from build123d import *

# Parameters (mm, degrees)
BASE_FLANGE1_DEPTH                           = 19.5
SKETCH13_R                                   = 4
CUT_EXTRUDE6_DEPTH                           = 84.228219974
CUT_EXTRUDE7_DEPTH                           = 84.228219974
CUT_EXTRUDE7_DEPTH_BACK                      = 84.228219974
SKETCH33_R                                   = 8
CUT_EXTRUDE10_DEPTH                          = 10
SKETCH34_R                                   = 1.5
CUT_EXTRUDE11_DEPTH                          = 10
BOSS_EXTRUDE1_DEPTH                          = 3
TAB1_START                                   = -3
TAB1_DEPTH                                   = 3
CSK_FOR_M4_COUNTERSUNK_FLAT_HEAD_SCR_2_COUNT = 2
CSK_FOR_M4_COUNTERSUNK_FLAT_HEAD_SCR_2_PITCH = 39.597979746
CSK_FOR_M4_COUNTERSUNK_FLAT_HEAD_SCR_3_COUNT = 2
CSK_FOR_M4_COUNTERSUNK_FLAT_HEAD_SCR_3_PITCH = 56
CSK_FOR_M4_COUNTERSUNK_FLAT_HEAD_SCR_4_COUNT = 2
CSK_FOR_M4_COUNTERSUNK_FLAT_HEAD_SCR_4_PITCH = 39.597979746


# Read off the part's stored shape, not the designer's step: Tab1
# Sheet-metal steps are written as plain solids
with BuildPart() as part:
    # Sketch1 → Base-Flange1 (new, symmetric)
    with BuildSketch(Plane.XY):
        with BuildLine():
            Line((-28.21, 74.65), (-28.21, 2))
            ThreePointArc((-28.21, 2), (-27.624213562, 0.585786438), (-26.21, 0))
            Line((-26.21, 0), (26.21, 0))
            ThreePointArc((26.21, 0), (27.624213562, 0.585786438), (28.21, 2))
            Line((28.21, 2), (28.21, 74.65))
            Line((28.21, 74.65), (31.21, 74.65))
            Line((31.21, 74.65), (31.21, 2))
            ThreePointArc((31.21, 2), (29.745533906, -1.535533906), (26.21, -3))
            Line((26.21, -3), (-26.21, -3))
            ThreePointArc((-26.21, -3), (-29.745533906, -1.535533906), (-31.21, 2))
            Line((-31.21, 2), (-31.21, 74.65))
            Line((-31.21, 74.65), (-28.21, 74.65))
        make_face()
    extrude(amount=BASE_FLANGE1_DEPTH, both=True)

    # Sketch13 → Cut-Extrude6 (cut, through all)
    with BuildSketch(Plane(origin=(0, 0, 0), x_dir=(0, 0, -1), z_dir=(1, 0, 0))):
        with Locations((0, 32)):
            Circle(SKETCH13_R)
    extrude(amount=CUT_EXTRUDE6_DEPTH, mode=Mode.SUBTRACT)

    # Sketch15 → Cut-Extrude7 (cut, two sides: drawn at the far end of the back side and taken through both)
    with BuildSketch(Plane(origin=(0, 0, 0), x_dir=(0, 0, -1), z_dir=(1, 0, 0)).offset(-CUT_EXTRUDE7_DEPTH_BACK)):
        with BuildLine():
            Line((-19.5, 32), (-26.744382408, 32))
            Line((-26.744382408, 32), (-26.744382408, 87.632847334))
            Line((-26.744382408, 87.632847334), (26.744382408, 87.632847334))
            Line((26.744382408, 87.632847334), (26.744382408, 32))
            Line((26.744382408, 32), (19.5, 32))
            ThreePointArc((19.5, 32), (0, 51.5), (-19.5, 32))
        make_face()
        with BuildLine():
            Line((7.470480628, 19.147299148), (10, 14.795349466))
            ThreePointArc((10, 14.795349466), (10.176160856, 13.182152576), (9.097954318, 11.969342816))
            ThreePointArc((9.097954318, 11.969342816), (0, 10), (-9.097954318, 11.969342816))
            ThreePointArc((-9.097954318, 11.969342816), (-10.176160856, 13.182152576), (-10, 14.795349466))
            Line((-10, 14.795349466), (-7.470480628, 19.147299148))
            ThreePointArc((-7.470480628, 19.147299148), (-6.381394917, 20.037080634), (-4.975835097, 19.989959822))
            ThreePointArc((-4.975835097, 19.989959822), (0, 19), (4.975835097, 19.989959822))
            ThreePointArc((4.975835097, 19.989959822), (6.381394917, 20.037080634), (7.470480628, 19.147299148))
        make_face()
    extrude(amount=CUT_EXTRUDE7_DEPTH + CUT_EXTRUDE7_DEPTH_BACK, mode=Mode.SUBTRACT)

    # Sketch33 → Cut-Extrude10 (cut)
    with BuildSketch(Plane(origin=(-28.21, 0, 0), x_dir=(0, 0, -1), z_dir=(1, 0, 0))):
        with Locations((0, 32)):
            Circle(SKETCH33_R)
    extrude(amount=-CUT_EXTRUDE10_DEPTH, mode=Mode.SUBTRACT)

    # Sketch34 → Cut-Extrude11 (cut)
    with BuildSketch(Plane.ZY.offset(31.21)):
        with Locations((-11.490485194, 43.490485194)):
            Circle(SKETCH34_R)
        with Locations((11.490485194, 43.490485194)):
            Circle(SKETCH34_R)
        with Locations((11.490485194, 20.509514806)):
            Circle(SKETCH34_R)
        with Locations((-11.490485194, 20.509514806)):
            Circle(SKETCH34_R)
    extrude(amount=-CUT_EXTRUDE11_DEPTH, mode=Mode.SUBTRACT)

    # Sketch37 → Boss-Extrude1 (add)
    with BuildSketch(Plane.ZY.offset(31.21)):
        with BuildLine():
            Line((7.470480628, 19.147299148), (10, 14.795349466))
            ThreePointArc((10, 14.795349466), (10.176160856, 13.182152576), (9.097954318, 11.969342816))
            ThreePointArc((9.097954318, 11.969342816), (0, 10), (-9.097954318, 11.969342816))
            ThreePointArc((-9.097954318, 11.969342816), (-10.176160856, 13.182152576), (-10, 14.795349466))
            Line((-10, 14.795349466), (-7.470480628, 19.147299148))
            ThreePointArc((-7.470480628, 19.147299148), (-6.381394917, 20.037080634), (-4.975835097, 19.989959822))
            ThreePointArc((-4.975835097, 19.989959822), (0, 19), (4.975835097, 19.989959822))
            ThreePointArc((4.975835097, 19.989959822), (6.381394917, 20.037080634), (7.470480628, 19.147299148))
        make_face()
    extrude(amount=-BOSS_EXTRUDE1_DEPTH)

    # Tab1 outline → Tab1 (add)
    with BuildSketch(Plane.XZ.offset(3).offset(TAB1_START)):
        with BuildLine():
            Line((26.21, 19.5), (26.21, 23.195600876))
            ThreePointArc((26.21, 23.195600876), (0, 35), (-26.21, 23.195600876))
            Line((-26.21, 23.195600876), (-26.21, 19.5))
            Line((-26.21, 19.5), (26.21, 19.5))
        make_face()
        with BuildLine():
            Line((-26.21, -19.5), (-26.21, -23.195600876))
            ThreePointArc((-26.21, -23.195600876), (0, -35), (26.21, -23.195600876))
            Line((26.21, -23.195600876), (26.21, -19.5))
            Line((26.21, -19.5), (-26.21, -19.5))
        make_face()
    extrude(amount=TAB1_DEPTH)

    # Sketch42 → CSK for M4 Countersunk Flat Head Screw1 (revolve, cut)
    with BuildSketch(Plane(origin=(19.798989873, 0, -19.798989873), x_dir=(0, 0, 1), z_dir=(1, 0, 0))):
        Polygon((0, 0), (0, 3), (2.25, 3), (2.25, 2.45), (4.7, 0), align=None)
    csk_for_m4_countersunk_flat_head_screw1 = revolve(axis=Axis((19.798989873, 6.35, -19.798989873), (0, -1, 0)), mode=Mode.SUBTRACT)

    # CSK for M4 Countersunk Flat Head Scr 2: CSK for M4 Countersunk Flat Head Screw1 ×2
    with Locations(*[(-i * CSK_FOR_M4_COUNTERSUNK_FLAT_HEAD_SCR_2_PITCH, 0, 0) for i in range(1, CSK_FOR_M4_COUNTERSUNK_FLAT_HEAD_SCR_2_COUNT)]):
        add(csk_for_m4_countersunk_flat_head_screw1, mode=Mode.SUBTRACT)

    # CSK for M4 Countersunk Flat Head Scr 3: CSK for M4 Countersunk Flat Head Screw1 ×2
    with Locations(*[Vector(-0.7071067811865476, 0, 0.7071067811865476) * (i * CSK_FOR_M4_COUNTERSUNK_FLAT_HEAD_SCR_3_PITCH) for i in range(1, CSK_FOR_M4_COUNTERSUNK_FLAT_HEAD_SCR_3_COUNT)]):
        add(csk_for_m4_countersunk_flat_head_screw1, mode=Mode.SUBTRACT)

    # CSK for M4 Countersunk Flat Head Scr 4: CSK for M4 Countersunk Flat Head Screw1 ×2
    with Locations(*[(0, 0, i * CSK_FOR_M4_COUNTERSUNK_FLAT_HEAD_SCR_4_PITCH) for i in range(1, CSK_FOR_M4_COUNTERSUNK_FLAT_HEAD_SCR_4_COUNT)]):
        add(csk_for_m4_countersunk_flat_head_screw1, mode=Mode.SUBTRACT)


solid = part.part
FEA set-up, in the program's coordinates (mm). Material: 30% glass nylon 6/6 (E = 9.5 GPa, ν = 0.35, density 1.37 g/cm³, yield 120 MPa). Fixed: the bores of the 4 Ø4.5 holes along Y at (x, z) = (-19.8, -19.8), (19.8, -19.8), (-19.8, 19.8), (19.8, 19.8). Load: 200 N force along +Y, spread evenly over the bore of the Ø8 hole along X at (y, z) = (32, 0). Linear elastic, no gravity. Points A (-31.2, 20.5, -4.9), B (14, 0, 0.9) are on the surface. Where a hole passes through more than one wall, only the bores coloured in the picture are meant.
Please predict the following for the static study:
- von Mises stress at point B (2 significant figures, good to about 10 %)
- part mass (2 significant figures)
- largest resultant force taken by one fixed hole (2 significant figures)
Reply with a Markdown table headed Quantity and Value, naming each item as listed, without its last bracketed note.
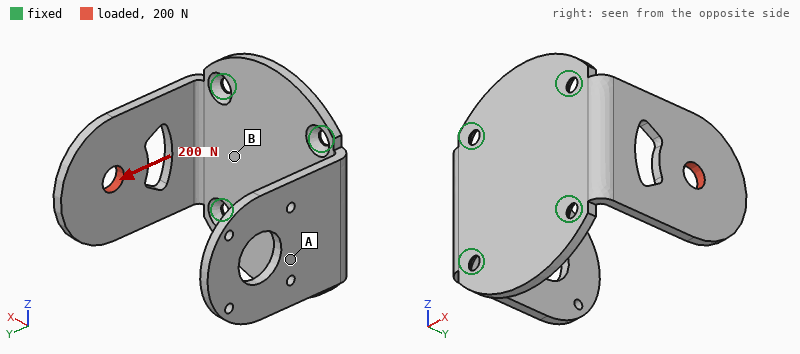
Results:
| Quantity | Value |
|---|---|
| von Mises stress at point B | 11 MPa |
| part mass | 27 g |
| largest resultant force taken by one fixed hole | 200 N |
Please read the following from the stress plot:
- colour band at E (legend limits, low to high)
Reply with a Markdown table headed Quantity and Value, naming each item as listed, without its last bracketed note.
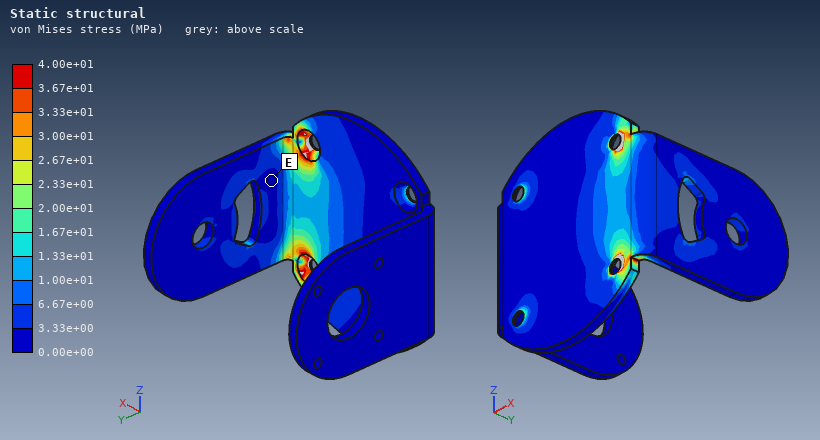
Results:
| Quantity | Value |
|---|---|
| colour band at E | 0.00e+00 to 3.33e+00 MPa |
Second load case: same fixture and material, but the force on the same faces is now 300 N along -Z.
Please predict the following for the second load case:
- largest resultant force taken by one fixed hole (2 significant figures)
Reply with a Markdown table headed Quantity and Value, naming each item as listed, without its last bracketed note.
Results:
| Quantity | Value |
|---|---|
| largest resultant force taken by one fixed hole | 390 N |
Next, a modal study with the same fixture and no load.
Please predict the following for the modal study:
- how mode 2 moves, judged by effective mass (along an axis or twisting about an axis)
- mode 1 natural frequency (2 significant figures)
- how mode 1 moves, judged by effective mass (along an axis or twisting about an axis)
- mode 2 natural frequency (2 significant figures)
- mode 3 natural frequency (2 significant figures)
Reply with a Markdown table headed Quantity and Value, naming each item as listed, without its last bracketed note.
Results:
| Quantity | Value |
|---|---|
| how mode 2 moves, judged by effective mass | along X |
| mode 1 natural frequency | 350 Hz |
| how mode 1 moves, judged by effective mass | along X |
| mode 2 natural frequency | 410 Hz |
| mode 3 natural frequency | 1200 Hz |
